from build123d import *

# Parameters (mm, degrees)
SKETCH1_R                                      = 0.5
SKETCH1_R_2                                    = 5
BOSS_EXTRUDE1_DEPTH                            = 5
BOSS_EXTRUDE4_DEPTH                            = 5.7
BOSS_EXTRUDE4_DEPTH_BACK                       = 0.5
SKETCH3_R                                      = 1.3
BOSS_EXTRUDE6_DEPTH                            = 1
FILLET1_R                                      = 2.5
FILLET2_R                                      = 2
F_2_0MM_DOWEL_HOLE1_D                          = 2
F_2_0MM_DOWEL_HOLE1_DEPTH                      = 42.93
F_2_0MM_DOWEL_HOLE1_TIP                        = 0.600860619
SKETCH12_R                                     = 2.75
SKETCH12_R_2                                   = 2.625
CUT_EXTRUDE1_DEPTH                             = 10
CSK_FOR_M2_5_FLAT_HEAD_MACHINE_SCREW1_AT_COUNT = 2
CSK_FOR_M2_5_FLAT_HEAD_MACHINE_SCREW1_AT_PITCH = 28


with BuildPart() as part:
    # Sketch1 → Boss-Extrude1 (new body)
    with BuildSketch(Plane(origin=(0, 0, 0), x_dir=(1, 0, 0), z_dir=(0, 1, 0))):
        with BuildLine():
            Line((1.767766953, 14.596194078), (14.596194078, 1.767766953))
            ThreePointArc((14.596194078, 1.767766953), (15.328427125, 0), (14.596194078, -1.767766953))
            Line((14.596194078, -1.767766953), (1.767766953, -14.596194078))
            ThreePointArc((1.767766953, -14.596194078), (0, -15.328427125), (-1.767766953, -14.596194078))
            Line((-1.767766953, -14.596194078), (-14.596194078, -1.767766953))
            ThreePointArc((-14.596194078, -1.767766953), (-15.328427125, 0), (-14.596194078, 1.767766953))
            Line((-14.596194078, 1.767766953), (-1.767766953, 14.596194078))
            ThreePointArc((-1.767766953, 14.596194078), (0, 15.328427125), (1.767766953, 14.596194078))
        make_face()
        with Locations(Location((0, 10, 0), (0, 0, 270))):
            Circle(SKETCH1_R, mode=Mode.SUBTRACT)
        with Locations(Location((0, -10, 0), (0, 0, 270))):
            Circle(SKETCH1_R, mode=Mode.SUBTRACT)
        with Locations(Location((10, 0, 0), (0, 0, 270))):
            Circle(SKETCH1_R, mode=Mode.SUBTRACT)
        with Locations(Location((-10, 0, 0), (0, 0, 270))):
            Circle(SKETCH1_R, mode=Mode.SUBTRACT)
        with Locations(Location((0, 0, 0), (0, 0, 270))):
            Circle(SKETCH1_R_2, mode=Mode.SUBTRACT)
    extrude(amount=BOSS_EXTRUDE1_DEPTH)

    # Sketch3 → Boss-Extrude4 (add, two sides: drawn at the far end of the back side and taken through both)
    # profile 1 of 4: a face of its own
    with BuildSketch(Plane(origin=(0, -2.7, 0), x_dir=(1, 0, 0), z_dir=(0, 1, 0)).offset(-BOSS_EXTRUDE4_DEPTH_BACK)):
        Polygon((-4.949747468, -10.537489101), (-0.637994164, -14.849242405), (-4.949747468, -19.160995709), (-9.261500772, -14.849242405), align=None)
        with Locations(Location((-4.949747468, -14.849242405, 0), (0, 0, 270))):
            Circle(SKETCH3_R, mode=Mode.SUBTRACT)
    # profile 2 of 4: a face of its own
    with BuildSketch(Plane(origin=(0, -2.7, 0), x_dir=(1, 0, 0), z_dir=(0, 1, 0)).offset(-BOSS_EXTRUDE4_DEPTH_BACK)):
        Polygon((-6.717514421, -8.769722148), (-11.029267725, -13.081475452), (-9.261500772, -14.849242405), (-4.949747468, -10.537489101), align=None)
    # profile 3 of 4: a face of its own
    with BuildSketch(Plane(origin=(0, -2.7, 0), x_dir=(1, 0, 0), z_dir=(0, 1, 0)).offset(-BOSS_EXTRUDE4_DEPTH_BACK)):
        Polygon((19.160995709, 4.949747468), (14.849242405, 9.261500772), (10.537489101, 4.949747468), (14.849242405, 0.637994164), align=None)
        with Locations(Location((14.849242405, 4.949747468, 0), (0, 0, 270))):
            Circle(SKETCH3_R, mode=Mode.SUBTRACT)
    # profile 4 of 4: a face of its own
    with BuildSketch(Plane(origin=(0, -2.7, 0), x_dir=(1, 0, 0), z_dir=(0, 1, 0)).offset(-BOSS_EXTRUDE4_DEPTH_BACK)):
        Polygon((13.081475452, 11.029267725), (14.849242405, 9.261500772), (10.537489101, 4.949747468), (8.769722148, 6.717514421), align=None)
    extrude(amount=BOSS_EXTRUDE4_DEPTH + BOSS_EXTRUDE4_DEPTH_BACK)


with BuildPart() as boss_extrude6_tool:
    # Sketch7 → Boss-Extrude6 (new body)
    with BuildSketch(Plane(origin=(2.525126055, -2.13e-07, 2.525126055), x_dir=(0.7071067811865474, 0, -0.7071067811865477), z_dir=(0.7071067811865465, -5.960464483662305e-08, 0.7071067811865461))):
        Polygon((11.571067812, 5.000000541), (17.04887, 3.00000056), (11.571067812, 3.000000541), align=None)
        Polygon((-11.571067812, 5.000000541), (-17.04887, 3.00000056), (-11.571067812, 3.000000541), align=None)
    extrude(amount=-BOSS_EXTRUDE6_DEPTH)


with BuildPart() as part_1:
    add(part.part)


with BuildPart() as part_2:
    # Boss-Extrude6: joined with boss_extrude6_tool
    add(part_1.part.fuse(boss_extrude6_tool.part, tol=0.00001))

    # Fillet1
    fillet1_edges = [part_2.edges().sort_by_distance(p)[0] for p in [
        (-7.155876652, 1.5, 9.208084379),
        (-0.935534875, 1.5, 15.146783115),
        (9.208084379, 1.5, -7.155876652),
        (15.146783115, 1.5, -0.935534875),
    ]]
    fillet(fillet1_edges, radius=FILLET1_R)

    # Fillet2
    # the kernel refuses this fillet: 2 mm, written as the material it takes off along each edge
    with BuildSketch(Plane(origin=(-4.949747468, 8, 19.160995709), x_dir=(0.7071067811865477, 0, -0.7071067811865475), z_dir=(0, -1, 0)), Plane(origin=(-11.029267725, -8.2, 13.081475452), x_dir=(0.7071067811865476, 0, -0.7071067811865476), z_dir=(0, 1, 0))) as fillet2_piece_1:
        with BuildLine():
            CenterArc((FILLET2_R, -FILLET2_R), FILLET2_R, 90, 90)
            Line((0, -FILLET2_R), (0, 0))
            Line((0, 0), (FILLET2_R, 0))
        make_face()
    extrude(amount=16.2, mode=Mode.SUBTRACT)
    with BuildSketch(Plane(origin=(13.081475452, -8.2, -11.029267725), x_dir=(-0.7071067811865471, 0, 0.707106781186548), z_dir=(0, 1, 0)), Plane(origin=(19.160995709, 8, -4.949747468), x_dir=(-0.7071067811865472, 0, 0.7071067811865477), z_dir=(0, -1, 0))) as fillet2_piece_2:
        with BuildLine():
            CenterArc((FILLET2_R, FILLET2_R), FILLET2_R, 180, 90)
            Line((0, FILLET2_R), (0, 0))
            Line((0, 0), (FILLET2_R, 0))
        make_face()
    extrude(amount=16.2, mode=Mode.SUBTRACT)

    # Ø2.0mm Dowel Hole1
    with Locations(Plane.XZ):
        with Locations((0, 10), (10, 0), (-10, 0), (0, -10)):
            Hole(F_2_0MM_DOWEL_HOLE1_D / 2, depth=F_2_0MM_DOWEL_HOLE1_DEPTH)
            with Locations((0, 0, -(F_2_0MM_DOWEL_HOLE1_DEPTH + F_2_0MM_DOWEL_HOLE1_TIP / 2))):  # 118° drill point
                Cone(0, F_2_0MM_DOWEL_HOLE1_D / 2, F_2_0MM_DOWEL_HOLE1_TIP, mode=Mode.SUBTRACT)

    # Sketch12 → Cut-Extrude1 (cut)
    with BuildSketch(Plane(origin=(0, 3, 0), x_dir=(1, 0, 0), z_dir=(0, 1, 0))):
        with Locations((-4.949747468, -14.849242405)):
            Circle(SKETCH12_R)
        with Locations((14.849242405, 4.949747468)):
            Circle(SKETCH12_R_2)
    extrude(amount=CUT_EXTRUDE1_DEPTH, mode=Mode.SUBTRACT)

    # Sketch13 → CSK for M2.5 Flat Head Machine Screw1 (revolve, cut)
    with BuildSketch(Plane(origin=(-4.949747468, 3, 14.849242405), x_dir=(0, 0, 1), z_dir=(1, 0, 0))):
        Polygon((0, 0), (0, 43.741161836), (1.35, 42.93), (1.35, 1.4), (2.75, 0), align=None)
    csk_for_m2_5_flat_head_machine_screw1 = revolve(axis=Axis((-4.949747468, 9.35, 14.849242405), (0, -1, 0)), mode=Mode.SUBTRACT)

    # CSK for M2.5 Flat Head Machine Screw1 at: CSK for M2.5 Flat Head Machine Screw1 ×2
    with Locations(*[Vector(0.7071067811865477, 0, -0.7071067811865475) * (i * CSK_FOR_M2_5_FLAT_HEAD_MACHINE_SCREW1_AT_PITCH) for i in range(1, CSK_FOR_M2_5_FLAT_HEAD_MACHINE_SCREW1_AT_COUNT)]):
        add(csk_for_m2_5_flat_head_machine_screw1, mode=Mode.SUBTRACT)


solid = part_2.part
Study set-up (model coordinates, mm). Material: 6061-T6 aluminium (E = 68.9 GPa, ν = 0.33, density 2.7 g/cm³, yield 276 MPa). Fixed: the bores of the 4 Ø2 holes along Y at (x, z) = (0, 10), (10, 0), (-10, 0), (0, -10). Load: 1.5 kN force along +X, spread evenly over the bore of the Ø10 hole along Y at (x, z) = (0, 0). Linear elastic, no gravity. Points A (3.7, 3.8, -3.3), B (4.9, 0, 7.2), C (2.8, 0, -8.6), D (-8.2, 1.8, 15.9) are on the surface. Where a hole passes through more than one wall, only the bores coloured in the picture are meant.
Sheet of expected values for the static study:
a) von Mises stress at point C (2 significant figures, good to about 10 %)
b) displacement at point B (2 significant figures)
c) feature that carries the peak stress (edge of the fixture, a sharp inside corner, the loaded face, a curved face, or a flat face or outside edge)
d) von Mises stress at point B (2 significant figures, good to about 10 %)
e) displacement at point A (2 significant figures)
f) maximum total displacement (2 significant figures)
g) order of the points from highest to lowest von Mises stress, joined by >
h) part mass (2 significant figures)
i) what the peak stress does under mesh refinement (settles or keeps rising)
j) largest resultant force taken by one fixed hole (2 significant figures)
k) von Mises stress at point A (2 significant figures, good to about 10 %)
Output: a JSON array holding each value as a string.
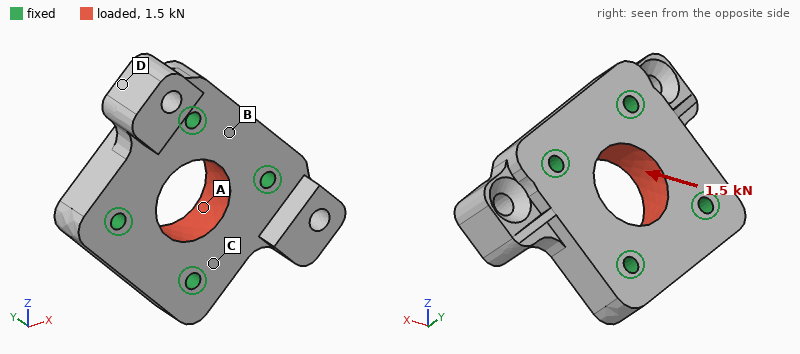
["8.4 MPa", "1.0 µm", "edge of the fixture", "5.2 MPa", "1.5 µm", "1.6 µm", "A > C > B > D", "7.3 g", "keeps rising", "450 N", "14 MPa"]
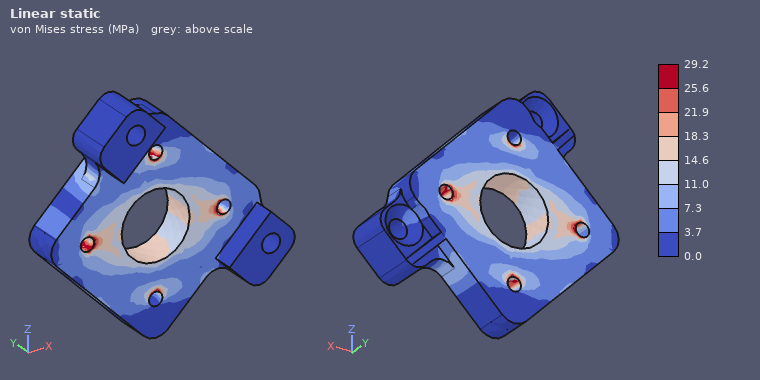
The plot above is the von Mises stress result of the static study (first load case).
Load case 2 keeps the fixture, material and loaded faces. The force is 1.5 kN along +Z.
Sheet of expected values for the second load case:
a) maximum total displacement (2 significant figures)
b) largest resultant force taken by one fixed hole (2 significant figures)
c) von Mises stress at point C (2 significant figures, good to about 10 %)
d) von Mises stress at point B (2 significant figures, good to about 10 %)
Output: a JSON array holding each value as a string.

["1.6 µm", "450 N", "8.9 MPa", "7.0 MPa"]
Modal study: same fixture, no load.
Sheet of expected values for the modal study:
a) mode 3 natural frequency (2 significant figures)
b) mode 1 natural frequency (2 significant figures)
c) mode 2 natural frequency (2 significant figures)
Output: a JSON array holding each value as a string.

["47 kHz", "28 kHz", "28 kHz"]
